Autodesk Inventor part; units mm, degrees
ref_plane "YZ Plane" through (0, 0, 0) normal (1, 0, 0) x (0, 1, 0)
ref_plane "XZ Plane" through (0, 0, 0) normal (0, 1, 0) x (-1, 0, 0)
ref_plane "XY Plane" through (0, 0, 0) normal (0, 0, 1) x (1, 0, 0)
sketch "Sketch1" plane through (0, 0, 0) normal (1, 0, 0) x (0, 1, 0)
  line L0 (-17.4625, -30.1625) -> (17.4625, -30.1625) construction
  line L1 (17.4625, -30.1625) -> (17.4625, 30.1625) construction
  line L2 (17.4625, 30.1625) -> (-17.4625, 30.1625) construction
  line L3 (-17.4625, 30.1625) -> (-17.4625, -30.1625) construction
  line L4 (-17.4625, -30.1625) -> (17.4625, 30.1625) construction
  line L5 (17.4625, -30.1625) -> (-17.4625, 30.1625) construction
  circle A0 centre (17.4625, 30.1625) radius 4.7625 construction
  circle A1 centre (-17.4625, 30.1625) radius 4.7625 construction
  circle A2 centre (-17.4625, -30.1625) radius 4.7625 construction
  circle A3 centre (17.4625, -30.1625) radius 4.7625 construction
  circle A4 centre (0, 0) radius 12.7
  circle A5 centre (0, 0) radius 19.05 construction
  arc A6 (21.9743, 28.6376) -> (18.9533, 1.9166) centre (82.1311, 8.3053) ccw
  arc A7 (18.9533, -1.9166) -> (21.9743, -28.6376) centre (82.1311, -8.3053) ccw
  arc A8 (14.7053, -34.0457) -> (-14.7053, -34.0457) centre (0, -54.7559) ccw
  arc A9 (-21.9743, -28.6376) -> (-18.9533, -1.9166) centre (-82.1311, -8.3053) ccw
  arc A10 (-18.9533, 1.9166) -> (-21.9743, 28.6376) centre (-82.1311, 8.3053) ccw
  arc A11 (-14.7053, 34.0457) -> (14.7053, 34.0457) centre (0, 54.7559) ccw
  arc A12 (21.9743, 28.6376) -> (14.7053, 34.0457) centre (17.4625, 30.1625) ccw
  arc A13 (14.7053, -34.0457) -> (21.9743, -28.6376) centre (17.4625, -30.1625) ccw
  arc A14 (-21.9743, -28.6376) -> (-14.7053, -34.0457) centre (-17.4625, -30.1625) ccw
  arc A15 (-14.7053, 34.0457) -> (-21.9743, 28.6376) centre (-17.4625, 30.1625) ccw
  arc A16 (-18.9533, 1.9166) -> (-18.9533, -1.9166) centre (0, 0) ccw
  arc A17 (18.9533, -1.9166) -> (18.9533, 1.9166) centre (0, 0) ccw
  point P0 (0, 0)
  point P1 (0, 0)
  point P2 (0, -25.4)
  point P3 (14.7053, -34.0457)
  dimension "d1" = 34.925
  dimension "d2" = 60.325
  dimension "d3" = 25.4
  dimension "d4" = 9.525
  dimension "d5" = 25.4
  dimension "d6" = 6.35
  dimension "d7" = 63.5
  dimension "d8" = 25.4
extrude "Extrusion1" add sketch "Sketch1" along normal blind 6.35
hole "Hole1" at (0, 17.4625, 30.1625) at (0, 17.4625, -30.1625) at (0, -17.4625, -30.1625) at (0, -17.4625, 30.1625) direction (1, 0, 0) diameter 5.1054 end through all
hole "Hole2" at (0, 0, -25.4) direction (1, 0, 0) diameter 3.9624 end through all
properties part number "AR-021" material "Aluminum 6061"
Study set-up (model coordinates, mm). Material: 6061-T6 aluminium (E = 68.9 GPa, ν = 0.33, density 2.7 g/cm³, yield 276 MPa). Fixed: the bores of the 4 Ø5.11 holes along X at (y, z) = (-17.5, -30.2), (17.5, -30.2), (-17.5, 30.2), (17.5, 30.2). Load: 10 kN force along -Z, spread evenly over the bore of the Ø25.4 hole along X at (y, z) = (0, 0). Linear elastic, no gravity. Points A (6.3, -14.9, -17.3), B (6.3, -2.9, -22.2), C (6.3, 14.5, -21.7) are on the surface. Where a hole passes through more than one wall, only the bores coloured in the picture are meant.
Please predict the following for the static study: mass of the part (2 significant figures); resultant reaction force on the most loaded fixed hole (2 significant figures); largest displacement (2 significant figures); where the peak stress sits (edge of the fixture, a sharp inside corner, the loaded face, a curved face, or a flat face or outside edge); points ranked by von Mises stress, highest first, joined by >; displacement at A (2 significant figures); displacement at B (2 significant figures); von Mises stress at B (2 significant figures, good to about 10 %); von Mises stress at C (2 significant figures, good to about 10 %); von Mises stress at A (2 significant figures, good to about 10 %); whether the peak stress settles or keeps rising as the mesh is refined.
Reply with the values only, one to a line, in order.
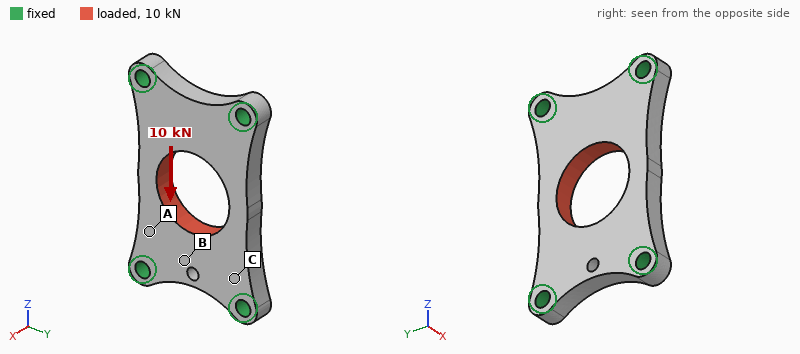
33 g
2.7 kN
11 µm
edge of the fixture
C > A > B
5.8 µm
9.1 µm
13 MPa
33 MPa
27 MPa
keeps rising
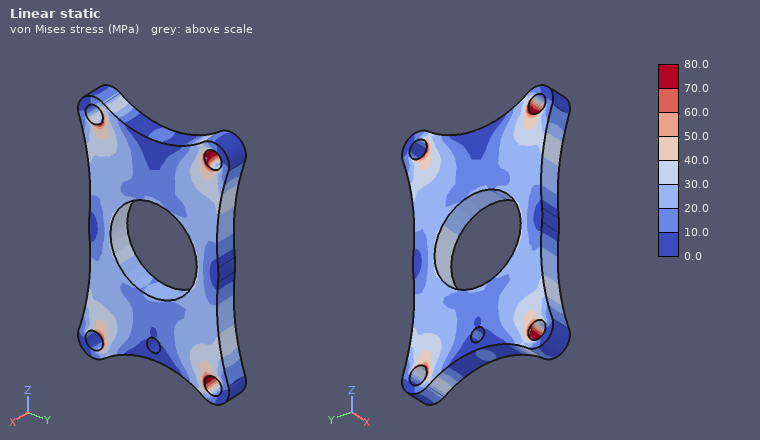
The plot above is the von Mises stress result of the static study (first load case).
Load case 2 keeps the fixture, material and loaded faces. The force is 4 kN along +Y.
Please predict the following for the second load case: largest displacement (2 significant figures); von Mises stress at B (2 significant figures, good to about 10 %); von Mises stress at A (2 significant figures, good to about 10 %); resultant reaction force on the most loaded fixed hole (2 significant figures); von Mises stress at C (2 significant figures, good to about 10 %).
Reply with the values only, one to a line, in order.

15 µm
15 MPa
7.4 MPa
1.3 kN
12 MPa
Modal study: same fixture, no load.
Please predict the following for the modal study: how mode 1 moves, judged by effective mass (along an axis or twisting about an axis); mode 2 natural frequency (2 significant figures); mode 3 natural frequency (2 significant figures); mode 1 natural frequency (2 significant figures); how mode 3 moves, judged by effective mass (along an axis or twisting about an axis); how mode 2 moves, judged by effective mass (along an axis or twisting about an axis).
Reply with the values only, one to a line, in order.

along X
12 kHz
16 kHz
8900 Hz
twisting about Y
twisting about Z
